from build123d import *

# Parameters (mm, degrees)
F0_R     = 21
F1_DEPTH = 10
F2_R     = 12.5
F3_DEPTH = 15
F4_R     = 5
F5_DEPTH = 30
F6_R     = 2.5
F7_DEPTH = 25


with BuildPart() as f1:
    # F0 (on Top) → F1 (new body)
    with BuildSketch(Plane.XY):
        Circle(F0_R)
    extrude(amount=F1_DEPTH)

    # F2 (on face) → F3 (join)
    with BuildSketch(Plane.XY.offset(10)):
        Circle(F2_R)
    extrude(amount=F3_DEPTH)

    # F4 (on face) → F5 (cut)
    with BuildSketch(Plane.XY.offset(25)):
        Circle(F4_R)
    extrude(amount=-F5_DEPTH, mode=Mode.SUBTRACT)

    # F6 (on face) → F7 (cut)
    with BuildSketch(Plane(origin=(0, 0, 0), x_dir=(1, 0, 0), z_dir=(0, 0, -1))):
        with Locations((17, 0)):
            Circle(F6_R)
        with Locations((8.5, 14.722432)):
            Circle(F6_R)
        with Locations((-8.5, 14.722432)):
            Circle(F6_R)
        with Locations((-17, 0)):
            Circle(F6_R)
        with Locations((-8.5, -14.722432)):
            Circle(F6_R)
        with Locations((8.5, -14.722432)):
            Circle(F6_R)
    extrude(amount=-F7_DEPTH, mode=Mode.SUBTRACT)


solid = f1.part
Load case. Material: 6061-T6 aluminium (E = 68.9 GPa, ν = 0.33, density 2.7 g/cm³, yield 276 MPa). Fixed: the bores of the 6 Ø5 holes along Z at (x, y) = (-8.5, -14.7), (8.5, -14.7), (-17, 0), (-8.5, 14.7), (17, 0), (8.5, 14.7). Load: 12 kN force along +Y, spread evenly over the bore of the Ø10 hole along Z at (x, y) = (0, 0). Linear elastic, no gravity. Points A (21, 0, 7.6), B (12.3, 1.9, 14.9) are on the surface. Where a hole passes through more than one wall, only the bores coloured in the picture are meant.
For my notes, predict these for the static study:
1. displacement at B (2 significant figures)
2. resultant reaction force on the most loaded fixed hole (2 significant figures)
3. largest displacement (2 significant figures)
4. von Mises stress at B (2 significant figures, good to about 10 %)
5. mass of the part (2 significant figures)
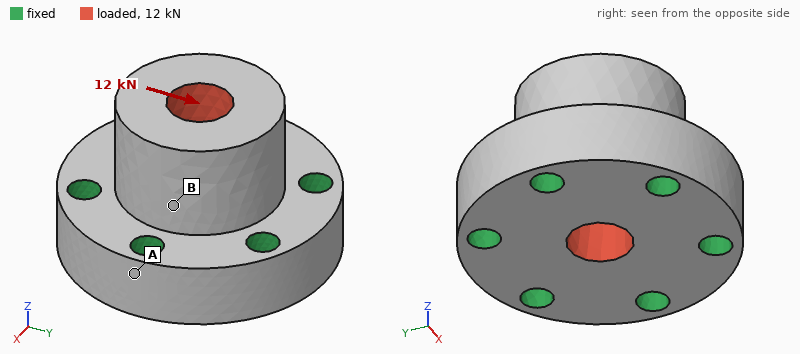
7.6 µm
3.1 kN
19 µm
23 MPa
49 g
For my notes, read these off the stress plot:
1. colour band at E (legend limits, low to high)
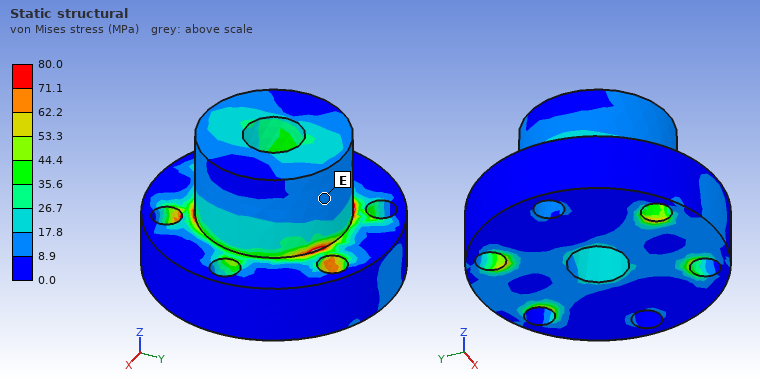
8.9 to 17.8 MPa
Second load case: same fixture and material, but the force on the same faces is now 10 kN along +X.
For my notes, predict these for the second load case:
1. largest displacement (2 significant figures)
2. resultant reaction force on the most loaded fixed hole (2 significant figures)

16 µm
3.0 kN
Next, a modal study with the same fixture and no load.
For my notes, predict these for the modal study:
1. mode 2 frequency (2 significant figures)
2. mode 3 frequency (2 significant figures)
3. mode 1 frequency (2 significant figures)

29 kHz
43 kHz
29 kHz
